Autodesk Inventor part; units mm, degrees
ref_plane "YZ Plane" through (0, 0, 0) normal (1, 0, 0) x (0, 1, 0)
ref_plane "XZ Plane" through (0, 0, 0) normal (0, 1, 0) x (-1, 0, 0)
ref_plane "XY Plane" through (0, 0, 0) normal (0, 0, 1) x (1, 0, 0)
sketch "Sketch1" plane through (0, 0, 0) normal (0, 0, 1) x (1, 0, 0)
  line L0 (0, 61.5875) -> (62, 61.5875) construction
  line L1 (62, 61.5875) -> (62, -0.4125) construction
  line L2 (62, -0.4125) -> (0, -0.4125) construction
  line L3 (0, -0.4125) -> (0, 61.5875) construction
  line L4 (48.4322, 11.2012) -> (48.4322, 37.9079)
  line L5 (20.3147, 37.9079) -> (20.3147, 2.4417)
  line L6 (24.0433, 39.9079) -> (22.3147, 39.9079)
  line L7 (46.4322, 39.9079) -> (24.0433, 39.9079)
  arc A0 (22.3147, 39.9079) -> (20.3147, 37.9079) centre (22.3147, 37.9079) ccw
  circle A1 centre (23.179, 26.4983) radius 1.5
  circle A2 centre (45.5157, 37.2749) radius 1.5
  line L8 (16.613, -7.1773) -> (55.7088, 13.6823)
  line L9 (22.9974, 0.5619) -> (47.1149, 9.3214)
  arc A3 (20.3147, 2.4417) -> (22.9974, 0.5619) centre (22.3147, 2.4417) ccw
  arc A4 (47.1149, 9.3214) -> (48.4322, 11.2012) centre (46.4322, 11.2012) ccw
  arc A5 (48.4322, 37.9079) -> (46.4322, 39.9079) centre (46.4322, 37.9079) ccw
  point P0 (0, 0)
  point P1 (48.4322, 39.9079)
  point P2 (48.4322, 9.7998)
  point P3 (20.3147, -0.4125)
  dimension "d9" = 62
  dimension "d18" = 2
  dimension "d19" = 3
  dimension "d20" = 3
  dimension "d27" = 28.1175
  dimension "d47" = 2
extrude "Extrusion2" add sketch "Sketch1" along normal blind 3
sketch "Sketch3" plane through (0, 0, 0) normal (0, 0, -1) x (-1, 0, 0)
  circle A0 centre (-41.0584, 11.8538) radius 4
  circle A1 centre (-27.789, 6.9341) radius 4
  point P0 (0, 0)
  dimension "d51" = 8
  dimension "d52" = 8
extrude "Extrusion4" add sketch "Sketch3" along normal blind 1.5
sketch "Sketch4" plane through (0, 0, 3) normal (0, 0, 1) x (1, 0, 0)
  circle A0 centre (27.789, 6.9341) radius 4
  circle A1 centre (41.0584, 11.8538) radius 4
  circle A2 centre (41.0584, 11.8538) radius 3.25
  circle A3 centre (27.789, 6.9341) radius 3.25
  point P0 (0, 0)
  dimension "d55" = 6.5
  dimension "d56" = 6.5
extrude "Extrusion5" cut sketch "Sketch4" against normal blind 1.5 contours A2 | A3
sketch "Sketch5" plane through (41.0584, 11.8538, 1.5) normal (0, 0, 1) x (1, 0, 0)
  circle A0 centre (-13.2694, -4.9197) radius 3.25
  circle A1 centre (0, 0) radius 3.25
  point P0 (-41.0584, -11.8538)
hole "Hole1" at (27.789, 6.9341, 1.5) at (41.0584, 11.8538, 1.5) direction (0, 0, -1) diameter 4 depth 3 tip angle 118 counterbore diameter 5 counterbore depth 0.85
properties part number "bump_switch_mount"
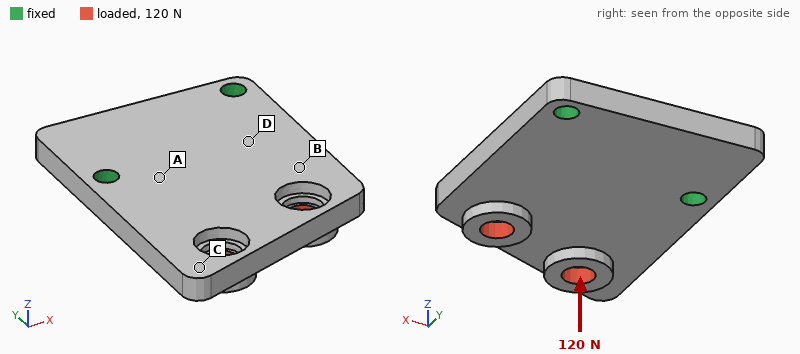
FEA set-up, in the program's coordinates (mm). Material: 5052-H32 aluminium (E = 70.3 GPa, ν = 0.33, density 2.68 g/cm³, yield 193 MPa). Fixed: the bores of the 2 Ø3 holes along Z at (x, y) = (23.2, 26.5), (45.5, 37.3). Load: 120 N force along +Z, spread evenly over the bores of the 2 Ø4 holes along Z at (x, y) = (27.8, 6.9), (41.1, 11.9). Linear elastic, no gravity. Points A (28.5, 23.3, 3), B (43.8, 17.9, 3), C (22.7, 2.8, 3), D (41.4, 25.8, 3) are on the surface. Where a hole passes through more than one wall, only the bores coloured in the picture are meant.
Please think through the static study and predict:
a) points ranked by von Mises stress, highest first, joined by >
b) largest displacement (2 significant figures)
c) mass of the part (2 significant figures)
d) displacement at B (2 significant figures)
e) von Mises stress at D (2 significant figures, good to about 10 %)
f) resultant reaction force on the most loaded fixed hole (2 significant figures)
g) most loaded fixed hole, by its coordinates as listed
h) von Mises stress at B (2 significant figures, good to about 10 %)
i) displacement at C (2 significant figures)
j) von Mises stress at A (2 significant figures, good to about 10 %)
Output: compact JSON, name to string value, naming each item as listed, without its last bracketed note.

{"points ranked by von Mises stress, highest first, joined by >": "A > D > B > C", "largest displacement": "0.12 mm", "mass of the part": "7.7 g", "displacement at B": "0.059 mm", "von Mises stress at D": "28 MPa", "resultant reaction force on the most loaded fixed hole": "110 N", "most loaded fixed hole, by its coordinates as listed": "(23.2, 26.5)", "von Mises stress at B": "19 MPa", "displacement at C": "0.11 mm", "von Mises stress at A": "44 MPa"}
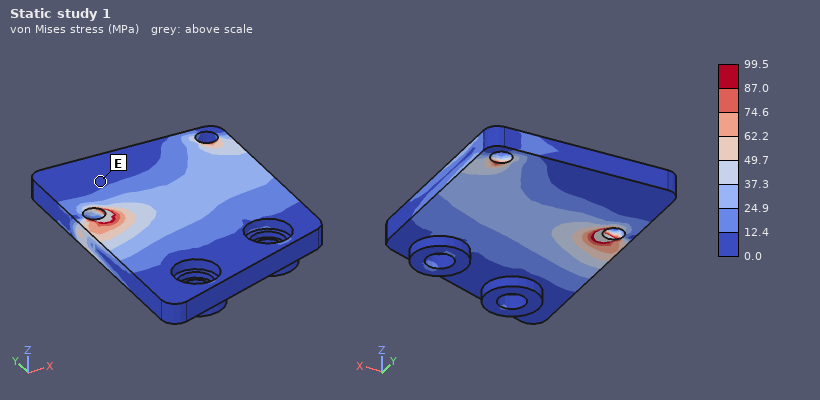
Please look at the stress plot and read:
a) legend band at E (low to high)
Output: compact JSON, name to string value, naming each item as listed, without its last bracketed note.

{"legend band at E": "0.0 to 12.4 MPa"}
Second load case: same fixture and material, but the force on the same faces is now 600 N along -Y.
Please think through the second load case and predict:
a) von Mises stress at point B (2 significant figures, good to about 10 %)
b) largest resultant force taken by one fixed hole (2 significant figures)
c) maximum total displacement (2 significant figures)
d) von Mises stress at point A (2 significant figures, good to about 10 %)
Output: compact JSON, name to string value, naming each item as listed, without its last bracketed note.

{"von Mises stress at point B": "17 MPa", "largest resultant force taken by one fixed hole": "310 N", "maximum total displacement": "90 µm", "von Mises stress at point A": "22 MPa"}
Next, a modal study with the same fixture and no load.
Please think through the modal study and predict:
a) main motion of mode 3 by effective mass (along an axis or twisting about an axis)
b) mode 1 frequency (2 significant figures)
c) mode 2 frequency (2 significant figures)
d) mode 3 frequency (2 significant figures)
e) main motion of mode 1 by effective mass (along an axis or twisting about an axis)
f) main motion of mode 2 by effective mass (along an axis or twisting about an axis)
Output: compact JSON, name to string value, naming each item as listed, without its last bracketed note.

{"main motion of mode 3 by effective mass": "along Z", "mode 1 frequency": "3700 Hz", "mode 2 frequency": "7500 Hz", "mode 3 frequency": "17 kHz", "main motion of mode 1 by effective mass": "along Z", "main motion of mode 2 by effective mass": "twisting about Y"}
